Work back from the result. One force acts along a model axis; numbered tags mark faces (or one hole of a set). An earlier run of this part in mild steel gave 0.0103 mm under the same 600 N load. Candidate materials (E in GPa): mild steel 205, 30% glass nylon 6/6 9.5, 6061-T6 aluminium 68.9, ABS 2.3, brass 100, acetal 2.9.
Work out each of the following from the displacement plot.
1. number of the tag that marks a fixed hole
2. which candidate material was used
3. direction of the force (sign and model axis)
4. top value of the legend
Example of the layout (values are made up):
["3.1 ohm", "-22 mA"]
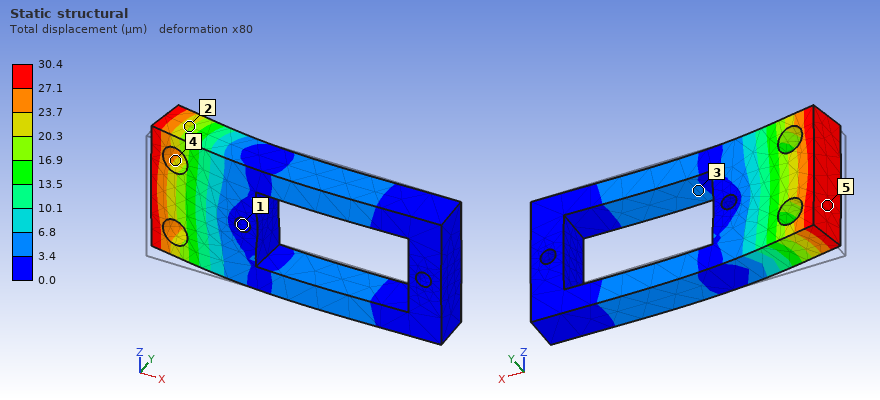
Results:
["1", "6061-T6 aluminium", "+Y", "30.4 µm"]
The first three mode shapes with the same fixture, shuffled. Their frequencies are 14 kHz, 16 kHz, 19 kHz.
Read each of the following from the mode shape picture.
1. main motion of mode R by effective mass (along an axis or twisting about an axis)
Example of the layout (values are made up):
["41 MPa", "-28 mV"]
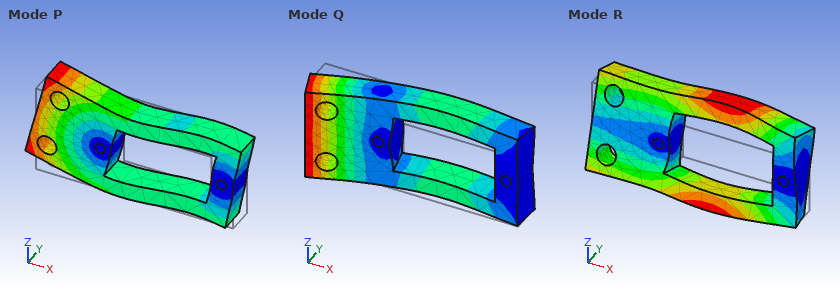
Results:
["twisting about X"]
